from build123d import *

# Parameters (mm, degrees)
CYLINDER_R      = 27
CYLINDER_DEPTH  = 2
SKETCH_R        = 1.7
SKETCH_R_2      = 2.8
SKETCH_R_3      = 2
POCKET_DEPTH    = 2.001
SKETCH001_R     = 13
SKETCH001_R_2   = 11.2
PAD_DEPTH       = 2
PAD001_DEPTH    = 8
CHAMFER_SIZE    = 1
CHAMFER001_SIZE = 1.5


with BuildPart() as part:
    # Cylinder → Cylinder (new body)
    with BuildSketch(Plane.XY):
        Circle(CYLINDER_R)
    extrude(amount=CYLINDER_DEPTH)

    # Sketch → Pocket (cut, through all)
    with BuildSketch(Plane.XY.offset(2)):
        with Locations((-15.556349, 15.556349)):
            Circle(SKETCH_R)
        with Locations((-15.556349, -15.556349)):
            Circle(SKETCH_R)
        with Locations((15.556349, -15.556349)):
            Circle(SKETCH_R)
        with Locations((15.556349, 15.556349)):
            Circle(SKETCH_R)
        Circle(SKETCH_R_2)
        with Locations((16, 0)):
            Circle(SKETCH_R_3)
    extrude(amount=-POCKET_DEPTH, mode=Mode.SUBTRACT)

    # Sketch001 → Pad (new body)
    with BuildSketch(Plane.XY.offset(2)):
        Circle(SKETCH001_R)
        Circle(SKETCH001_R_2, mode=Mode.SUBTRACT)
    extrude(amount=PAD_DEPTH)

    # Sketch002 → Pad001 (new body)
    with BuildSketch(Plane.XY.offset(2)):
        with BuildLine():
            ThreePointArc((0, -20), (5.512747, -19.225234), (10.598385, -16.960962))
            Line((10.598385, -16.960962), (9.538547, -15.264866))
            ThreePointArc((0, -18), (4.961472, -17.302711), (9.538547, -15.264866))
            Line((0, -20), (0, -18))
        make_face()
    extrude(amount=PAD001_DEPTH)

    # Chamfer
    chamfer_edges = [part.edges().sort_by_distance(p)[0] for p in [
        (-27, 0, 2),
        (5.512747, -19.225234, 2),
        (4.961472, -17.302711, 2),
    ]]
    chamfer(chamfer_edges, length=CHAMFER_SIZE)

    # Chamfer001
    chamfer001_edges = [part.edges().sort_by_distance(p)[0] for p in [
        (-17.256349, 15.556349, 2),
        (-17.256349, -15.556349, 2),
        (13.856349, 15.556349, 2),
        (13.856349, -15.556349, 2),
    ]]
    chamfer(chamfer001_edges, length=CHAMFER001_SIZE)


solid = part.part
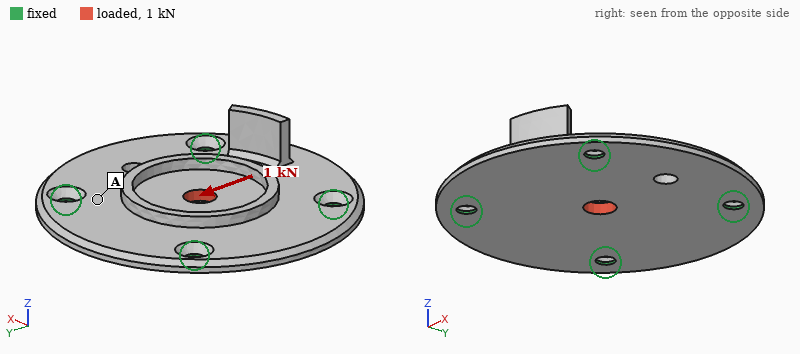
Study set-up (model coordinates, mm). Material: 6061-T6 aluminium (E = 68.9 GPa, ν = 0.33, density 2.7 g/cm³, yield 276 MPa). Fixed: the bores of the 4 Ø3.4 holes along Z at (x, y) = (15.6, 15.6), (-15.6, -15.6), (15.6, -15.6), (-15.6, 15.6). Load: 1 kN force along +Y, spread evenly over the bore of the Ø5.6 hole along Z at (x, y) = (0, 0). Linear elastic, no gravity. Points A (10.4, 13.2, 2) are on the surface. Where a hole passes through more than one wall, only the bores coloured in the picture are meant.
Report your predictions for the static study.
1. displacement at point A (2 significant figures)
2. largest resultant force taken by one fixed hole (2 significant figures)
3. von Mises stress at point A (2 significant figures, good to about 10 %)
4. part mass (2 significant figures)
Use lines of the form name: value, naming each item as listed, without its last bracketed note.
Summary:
displacement at point A: 2.7 µm
largest resultant force taken by one fixed hole: 260 N
von Mises stress at point A: 9.3 MPa
part mass: 13 g
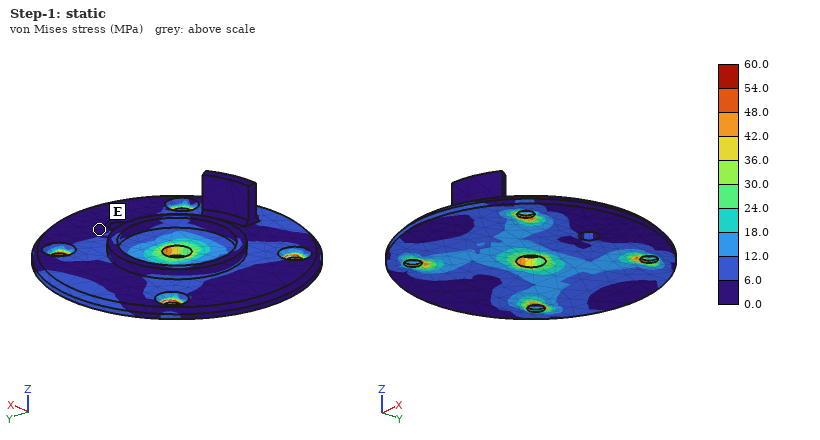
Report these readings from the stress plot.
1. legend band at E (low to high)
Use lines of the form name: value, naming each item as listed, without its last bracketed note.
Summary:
legend band at E: 0.0 to 6.0 MPa
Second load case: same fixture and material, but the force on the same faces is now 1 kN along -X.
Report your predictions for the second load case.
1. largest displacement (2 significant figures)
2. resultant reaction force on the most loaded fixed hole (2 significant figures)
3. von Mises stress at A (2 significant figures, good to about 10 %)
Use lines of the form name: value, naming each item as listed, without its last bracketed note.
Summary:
largest displacement: 6.3 µm
resultant reaction force on the most loaded fixed hole: 260 N
von Mises stress at A: 8.8 MPa
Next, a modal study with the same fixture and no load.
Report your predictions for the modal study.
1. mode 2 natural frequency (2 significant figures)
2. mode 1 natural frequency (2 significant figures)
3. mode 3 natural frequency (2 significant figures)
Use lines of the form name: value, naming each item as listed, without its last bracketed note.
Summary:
mode 2 natural frequency: 7400 Hz
mode 1 natural frequency: 6700 Hz
mode 3 natural frequency: 7400 Hz
